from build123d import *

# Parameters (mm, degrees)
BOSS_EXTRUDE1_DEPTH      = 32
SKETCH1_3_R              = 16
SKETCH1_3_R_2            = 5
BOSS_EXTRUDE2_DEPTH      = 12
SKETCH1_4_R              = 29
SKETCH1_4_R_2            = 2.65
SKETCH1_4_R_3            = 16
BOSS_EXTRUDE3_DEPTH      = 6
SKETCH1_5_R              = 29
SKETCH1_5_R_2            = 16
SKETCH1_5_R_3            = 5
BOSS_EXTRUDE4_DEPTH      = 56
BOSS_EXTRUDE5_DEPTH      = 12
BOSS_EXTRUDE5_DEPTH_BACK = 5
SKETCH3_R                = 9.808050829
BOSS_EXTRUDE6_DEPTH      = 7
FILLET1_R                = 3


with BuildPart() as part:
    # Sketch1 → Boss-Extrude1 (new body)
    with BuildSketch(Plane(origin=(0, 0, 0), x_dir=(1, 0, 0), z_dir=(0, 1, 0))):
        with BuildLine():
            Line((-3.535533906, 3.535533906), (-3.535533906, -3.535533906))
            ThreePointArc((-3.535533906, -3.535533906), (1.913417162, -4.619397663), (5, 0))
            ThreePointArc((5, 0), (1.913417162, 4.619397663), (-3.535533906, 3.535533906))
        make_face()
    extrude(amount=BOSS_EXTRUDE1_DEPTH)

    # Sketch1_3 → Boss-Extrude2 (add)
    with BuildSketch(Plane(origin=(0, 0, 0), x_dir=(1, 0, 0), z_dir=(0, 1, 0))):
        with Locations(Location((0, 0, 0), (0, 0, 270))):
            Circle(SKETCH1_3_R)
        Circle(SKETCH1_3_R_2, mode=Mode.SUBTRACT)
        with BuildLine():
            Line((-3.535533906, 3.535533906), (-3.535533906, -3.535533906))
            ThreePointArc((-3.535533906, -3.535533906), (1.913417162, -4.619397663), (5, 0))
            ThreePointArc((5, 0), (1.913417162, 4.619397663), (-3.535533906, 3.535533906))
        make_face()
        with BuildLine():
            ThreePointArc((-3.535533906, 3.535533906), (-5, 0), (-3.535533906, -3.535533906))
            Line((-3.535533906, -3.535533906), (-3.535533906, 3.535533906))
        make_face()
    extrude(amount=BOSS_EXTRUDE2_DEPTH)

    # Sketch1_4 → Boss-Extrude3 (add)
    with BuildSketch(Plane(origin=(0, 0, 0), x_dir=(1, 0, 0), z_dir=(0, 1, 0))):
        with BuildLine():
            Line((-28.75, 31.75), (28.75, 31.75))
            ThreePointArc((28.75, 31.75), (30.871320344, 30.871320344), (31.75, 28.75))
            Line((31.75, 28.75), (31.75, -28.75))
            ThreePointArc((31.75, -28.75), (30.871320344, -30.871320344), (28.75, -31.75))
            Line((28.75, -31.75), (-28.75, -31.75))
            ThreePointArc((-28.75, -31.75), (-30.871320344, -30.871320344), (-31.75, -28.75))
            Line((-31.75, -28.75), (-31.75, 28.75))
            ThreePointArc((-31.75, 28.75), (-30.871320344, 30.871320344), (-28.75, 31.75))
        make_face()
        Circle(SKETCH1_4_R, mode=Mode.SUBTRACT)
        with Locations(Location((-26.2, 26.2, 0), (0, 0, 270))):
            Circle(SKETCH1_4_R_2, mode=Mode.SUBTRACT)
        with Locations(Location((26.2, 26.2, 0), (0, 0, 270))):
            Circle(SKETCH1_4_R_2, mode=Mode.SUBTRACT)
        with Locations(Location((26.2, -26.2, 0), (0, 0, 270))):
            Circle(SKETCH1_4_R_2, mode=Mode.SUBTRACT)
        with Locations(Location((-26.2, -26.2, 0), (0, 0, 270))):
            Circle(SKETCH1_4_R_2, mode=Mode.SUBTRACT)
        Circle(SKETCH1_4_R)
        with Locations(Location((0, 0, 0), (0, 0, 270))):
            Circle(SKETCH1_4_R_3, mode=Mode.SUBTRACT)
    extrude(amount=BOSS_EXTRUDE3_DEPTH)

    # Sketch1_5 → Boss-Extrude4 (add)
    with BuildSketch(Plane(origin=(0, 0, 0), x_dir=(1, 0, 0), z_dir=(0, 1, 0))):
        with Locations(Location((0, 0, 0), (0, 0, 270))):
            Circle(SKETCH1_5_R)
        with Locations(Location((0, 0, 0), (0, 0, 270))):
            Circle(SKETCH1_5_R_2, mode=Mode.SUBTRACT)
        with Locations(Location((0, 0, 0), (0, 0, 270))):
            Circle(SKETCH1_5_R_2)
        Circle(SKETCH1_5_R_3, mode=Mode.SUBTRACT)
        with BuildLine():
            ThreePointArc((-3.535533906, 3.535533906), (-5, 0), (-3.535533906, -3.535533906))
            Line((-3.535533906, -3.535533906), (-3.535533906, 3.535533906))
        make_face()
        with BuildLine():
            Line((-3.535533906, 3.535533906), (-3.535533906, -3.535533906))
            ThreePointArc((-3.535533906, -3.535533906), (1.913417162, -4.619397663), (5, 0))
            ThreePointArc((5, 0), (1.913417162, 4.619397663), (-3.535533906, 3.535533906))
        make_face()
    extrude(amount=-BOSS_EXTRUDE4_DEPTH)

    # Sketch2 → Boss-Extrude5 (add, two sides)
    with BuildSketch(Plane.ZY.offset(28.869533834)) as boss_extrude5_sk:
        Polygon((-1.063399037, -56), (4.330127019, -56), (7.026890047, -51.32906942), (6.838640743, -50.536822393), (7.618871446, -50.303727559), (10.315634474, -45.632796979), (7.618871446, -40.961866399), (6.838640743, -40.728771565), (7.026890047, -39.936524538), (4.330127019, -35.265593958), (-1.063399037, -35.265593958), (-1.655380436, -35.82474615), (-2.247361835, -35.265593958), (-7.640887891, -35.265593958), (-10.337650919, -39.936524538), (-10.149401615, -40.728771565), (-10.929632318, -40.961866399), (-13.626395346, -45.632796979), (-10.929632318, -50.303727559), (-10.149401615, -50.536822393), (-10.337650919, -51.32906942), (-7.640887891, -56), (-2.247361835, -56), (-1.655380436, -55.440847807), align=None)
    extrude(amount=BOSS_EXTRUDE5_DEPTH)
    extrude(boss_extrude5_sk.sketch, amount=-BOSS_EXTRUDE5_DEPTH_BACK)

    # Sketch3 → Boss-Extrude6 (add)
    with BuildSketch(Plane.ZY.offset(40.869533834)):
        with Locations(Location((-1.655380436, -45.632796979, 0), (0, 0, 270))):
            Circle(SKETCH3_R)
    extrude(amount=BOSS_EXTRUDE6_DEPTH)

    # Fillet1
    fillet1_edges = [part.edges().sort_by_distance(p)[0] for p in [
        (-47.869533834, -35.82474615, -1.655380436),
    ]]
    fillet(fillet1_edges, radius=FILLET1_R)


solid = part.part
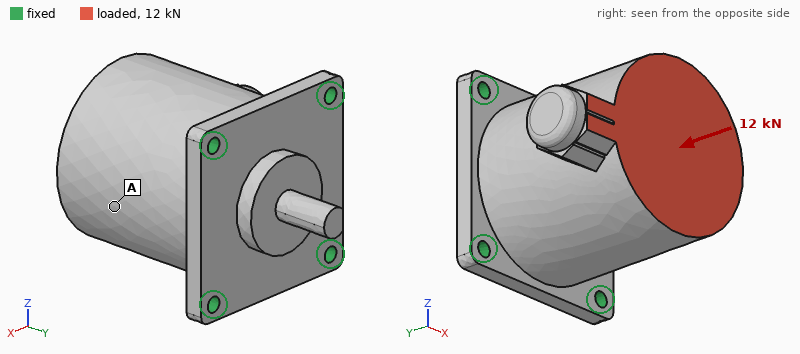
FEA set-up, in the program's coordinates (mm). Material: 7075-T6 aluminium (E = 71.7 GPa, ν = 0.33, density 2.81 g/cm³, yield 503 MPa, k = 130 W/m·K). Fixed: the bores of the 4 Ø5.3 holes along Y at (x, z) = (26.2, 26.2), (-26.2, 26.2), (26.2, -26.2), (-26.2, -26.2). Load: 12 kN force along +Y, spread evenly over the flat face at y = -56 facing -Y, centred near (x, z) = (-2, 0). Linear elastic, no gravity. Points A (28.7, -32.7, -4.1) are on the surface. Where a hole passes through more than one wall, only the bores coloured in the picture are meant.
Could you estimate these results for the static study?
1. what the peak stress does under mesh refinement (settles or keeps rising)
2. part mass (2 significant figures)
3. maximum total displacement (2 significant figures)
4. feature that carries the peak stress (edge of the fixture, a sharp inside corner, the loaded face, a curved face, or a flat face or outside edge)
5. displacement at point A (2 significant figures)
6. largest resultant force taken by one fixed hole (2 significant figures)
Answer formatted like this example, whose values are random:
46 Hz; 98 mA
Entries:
keeps rising; 520 g; 34 µm; edge of the fixture; 24 µm; 3.4 kN
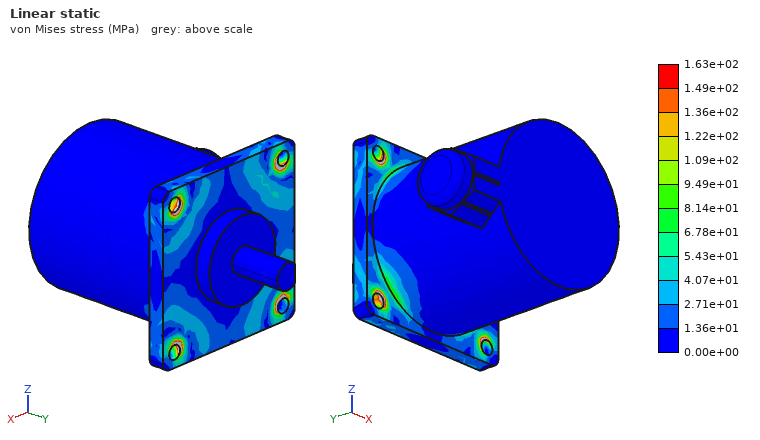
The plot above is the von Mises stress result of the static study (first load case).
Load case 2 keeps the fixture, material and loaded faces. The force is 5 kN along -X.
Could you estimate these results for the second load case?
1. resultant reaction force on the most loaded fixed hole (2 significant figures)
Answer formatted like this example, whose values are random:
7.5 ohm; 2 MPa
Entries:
3.5 kN
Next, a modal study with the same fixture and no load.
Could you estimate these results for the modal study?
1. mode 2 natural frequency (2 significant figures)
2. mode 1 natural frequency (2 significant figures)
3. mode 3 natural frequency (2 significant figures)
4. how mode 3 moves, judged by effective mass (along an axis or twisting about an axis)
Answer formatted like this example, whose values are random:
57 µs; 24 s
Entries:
3000 Hz; 2900 Hz; 4800 Hz; along Y
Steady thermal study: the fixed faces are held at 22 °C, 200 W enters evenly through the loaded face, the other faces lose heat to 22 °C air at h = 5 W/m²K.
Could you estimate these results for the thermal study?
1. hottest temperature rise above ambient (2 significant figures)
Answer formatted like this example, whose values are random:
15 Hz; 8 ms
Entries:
70 K
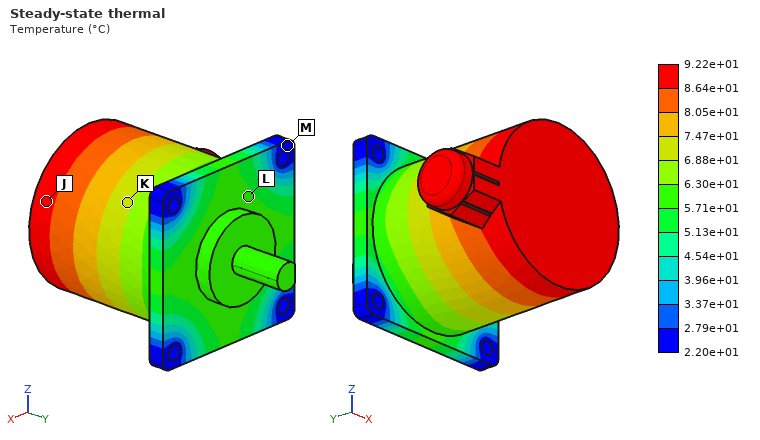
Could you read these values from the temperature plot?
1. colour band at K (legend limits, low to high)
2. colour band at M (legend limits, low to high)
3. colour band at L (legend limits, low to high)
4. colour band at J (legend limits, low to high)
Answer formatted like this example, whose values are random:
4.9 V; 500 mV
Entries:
6.88e+01 to 7.47e+01 °C; 2.20e+01 to 2.79e+01 °C; 5.71e+01 to 6.30e+01 °C; 8.64e+01 to 9.22e+01 °C
